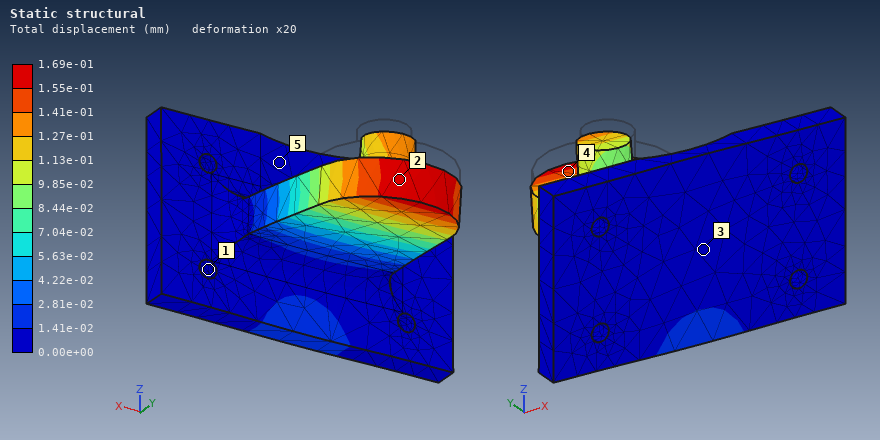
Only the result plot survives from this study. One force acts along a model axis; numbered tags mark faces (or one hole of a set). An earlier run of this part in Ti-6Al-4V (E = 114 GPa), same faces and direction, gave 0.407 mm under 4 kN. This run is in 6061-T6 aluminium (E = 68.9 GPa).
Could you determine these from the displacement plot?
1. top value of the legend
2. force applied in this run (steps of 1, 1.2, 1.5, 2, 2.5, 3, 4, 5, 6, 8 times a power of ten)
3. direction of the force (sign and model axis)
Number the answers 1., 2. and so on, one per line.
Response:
1. 1.69e-01 mm
2. 1 kN
3. -Z
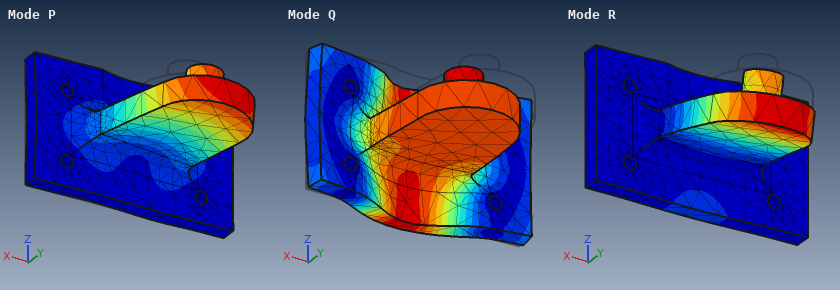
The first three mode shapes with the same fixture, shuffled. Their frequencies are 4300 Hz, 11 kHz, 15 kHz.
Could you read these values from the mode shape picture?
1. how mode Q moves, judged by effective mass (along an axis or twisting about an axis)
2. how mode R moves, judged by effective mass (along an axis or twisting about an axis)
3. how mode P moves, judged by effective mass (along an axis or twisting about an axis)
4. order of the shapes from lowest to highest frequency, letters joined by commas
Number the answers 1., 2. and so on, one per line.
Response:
1. along Y
2. along Z
3. along X
4. R, P, Q
